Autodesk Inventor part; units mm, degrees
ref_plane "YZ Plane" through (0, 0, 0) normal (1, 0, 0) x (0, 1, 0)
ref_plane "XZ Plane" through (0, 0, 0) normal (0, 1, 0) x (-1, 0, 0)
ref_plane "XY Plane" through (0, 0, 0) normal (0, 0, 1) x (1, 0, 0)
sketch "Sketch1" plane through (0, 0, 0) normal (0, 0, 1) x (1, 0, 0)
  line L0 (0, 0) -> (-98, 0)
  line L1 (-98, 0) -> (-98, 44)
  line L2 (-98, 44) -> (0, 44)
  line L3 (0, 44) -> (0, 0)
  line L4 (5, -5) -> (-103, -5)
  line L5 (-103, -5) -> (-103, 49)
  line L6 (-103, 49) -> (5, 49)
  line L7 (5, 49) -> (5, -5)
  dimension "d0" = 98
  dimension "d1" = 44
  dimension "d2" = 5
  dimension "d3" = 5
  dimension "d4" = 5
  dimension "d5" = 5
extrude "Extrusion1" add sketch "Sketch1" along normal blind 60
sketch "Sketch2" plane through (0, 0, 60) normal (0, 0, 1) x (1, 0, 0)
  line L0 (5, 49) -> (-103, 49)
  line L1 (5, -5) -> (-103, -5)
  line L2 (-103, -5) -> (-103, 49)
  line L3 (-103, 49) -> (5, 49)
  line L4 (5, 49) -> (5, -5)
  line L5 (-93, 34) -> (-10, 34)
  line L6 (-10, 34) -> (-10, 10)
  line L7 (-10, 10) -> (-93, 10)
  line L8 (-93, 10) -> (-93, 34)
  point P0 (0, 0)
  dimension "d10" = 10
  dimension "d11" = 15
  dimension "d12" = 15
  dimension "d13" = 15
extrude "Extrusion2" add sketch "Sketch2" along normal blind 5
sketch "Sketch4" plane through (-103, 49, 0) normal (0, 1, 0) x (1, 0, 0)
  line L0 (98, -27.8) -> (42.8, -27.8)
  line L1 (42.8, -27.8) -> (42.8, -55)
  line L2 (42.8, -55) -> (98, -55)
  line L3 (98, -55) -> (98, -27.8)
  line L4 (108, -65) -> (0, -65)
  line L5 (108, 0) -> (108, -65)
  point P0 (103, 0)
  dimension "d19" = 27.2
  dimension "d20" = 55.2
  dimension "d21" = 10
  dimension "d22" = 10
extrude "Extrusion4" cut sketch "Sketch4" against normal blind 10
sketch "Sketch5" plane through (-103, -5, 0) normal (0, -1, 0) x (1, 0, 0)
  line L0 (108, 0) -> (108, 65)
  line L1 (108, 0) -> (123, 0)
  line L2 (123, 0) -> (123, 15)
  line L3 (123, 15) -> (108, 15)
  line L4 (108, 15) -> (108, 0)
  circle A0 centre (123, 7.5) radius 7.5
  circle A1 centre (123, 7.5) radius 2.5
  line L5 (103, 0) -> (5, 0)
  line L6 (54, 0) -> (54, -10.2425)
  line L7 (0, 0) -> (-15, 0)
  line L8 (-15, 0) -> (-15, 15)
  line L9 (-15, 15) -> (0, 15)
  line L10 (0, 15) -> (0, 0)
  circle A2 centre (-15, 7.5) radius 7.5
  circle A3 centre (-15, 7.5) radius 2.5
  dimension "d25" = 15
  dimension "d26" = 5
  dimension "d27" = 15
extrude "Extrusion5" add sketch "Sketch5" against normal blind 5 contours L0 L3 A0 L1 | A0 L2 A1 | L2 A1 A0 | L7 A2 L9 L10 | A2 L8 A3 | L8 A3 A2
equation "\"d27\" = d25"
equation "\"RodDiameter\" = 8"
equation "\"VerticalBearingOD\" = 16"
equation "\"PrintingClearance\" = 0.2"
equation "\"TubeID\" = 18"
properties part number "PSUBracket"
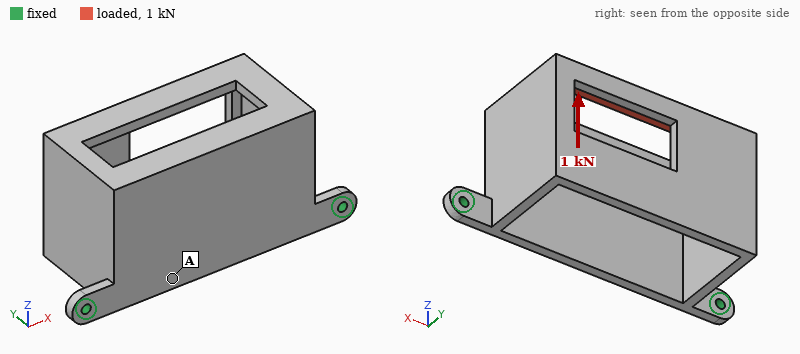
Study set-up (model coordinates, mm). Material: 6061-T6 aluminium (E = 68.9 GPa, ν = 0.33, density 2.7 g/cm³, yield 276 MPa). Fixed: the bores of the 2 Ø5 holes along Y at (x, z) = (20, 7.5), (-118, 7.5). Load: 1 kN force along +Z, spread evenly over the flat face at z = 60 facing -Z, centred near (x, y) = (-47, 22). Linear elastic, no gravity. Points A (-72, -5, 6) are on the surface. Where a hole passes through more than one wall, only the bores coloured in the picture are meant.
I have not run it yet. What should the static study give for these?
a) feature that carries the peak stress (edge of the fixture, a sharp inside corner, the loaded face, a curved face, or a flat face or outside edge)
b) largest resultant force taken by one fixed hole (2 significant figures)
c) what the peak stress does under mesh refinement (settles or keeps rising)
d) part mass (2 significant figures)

edge of the fixture
540 N
keeps rising
290 g
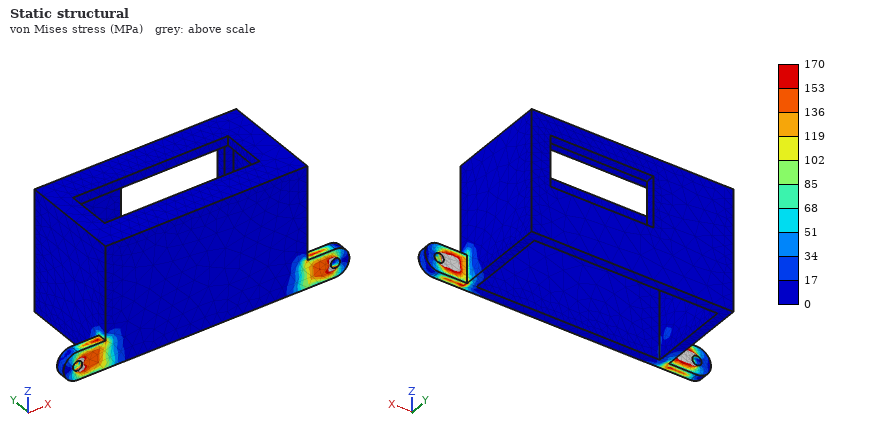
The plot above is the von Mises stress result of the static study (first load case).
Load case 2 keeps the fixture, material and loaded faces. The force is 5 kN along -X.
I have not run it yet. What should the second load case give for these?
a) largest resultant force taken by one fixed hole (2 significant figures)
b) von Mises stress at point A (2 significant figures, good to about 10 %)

3.4 kN
21 MPa
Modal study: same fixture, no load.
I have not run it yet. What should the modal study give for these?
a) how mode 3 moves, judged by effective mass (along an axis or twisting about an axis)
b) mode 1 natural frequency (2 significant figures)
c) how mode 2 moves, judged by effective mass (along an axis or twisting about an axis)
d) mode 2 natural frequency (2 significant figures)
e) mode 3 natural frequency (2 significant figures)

along Y
280 Hz
along X
880 Hz
1600 Hz
